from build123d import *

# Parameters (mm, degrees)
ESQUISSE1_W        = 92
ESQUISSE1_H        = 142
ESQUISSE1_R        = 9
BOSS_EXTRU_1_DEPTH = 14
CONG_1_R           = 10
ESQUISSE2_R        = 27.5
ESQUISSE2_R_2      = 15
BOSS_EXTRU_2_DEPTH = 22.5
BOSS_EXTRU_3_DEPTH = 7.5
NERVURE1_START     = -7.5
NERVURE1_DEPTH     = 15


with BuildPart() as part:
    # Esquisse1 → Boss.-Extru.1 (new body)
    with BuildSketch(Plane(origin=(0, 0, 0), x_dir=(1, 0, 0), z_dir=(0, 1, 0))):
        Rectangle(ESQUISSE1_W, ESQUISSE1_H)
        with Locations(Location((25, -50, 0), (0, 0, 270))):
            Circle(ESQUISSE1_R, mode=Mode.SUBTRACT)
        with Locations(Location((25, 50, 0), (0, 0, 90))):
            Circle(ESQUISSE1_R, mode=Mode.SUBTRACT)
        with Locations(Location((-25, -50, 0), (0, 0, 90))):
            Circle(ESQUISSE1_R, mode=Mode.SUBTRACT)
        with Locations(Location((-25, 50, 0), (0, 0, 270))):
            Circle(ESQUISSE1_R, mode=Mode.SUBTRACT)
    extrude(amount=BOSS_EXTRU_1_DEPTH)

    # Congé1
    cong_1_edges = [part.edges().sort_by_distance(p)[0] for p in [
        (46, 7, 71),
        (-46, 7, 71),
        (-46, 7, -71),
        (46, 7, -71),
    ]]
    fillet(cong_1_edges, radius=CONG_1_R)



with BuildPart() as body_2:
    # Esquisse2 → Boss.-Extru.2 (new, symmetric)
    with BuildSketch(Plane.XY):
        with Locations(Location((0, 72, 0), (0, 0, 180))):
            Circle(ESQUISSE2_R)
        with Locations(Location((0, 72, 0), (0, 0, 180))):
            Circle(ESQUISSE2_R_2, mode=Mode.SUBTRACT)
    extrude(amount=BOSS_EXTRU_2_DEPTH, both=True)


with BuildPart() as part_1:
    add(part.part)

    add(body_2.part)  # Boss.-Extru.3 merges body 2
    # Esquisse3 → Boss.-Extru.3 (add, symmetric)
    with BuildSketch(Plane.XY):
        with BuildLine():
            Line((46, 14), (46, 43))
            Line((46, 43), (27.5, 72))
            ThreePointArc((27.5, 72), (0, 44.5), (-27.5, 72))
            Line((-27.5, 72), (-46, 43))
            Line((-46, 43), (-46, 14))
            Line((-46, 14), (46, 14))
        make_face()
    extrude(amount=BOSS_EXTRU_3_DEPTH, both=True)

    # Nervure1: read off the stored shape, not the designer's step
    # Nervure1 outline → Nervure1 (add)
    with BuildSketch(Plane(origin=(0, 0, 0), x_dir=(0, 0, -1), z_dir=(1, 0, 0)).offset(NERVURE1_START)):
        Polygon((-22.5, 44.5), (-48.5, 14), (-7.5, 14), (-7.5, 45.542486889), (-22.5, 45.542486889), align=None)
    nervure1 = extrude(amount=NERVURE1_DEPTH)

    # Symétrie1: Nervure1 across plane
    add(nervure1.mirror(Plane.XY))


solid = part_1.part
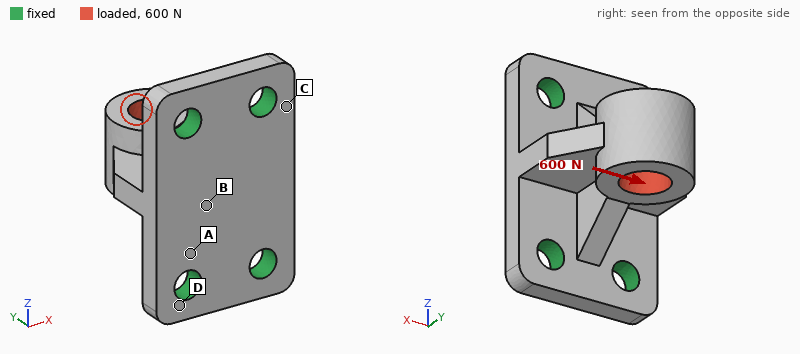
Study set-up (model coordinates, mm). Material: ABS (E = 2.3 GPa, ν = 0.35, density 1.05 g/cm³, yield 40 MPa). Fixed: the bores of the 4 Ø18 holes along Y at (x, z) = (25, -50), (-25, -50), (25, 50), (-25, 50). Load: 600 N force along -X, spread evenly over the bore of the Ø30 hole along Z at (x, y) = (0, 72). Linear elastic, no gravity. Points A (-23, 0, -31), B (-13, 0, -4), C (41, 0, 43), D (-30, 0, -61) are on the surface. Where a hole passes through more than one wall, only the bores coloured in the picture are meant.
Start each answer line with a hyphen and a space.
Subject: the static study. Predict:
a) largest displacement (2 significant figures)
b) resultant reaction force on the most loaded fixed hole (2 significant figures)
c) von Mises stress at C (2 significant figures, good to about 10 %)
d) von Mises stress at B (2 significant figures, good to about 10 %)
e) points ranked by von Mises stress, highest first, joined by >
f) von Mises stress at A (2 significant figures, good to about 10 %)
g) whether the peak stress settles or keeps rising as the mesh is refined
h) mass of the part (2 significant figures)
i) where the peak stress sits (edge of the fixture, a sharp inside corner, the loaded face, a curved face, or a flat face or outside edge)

- 0.35 mm
- 400 N
- 2.3 MPa
- 1.00 MPa
- C > A > B > D
- 1.5 MPa
- keeps rising
- 340 g
- edge of the fixture
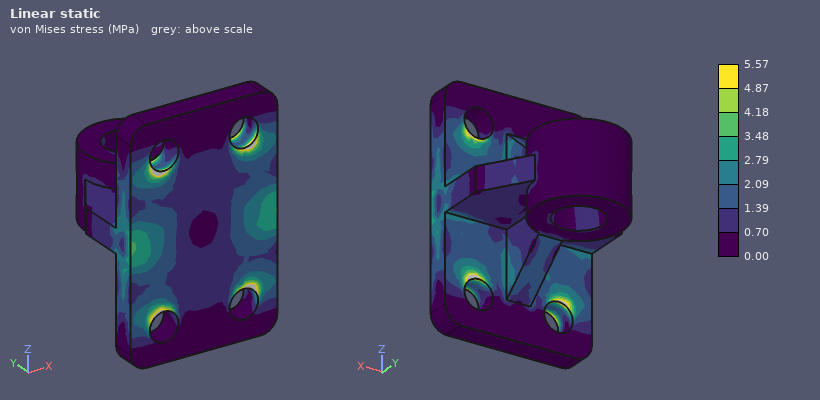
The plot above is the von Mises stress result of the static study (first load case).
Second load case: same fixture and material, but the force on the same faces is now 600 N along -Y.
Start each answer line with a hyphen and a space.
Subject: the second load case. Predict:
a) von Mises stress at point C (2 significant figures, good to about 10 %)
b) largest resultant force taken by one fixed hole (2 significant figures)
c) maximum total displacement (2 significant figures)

- 0.48 MPa
- 160 N
- 41 µm
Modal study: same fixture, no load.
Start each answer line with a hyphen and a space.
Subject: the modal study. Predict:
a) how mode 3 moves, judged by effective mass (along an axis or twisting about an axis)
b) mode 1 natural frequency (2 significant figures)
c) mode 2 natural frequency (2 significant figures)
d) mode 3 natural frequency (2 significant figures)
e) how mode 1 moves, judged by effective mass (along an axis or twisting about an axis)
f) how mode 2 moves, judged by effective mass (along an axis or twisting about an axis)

- along Y
- 730 Hz
- 1000 Hz
- 1600 Hz
- along X
- along Z
